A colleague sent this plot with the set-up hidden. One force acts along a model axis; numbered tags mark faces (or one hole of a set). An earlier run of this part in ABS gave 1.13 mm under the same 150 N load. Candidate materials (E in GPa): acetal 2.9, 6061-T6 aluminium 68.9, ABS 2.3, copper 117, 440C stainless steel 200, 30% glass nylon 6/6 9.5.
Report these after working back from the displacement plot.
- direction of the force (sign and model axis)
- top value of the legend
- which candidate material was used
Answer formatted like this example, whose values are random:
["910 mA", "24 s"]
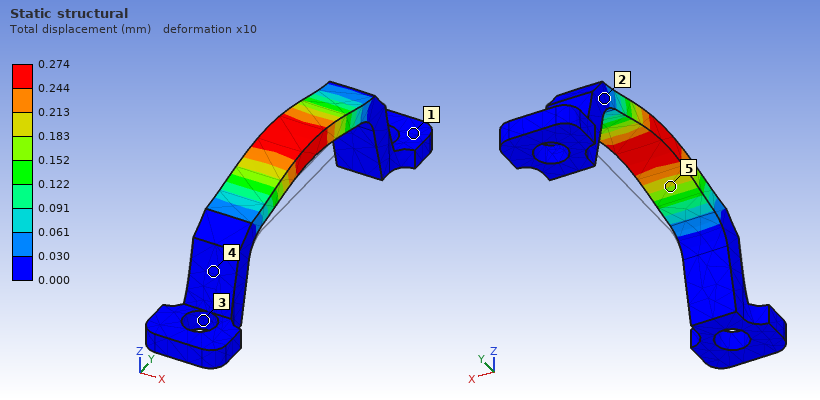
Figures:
["+Z", "0.274 mm", "30% glass nylon 6/6"]
